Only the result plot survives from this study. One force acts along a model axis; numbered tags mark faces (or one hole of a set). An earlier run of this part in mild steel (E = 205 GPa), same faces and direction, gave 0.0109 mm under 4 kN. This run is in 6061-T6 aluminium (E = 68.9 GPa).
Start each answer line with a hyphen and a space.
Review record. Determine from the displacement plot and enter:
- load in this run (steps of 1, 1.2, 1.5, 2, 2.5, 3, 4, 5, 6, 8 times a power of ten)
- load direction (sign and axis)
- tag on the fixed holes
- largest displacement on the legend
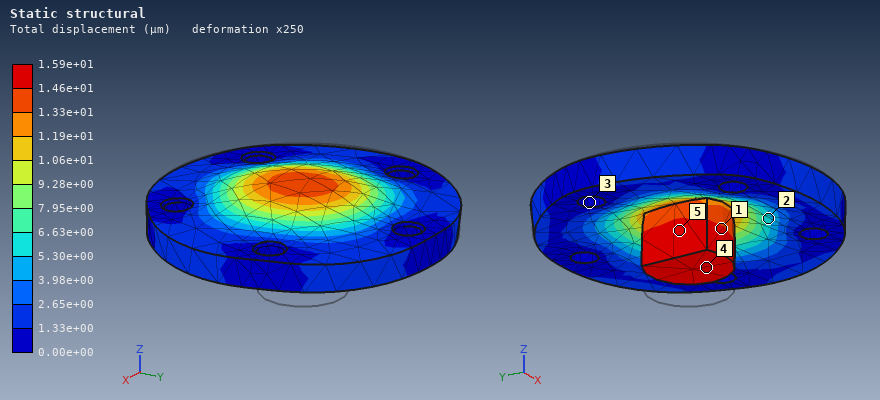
- 2 kN
- +Z
- 3
- 1.59e+01 µm
